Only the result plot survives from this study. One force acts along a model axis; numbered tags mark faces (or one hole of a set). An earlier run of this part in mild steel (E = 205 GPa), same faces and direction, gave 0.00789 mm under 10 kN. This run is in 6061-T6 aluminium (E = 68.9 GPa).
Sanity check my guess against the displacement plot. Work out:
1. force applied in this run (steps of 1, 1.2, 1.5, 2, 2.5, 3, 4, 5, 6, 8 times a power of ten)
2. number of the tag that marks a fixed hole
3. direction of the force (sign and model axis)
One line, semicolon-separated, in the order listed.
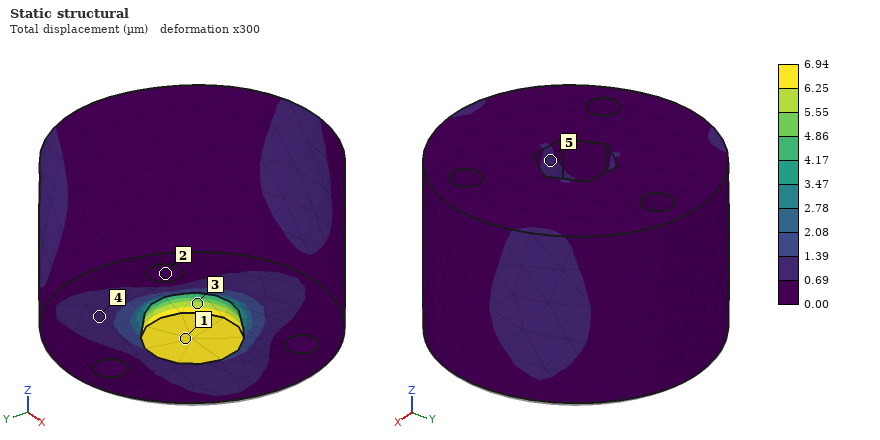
3 kN; 2; +Z
